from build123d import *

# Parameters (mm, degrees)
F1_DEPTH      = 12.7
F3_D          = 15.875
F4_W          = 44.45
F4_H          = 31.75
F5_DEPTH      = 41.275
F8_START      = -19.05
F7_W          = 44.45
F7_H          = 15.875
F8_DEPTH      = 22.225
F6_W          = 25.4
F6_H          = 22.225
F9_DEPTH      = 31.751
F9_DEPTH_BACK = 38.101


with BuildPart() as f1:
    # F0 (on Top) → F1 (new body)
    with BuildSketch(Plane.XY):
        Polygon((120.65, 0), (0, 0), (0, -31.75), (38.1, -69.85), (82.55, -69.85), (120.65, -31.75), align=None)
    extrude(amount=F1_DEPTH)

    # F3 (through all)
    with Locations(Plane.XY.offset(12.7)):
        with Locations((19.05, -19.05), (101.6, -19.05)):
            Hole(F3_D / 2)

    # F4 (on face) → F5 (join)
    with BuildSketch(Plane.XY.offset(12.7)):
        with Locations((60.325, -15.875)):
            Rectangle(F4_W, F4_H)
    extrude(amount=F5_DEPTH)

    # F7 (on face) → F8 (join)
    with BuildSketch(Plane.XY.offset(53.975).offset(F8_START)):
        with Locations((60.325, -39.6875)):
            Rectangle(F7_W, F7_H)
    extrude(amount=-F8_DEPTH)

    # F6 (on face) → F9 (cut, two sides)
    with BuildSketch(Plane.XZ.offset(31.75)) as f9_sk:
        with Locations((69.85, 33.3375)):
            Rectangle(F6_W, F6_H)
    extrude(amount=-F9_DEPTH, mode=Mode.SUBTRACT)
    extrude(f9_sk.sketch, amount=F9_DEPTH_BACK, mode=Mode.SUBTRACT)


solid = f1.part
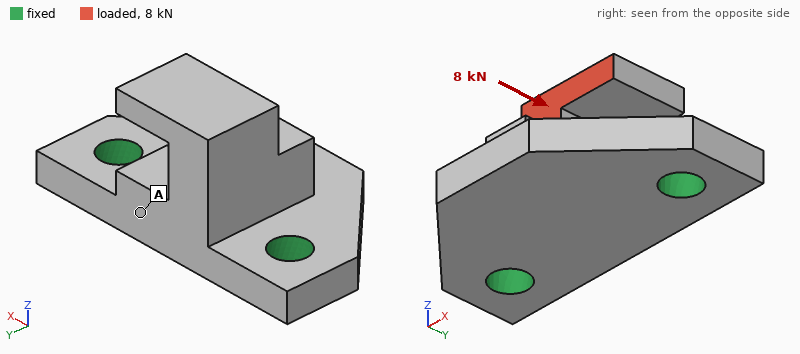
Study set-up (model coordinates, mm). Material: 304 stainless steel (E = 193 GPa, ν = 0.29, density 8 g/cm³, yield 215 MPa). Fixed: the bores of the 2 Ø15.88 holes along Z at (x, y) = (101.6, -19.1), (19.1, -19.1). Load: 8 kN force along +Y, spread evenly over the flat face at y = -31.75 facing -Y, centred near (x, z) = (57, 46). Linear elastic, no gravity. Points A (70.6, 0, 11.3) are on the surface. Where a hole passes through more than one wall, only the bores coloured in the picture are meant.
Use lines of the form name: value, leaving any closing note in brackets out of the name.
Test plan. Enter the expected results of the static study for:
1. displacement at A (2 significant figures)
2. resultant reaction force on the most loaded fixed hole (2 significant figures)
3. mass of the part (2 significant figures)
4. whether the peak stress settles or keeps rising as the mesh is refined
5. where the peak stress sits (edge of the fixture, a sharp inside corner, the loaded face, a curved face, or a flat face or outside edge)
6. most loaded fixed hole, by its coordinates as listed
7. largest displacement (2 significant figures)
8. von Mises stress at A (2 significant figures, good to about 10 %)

displacement at A: 21 µm
resultant reaction force on the most loaded fixed hole: 4.6 kN
mass of the part: 1.1 kg
whether the peak stress settles or keeps rising as the mesh is refined: keeps rising
where the peak stress sits: edge of the fixture
most loaded fixed hole, by its coordinates as listed: (19.1, -19.1)
largest displacement: 90 µm
von Mises stress at A: 25 MPa
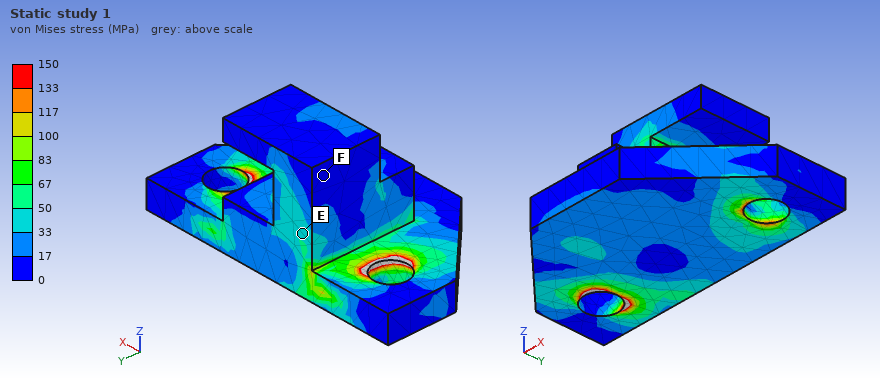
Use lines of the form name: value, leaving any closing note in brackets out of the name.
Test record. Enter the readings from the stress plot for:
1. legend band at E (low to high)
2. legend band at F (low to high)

legend band at E: 33 to 50 MPa
legend band at F: 0 to 17 MPa
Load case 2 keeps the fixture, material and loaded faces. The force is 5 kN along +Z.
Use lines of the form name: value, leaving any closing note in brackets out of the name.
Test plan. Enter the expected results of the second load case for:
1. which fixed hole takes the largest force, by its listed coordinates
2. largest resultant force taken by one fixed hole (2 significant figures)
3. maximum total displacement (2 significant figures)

which fixed hole takes the largest force, by its listed coordinates: (19.1, -19.1)
largest resultant force taken by one fixed hole: 3.0 kN
maximum total displacement: 57 µm
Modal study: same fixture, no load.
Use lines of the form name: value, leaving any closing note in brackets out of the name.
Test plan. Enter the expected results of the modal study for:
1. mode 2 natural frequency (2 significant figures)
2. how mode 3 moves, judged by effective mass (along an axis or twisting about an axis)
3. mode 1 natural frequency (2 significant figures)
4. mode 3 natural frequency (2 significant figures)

mode 2 natural frequency: 4600 Hz
how mode 3 moves, judged by effective mass: along Z
mode 1 natural frequency: 3300 Hz
mode 3 natural frequency: 6600 Hz
